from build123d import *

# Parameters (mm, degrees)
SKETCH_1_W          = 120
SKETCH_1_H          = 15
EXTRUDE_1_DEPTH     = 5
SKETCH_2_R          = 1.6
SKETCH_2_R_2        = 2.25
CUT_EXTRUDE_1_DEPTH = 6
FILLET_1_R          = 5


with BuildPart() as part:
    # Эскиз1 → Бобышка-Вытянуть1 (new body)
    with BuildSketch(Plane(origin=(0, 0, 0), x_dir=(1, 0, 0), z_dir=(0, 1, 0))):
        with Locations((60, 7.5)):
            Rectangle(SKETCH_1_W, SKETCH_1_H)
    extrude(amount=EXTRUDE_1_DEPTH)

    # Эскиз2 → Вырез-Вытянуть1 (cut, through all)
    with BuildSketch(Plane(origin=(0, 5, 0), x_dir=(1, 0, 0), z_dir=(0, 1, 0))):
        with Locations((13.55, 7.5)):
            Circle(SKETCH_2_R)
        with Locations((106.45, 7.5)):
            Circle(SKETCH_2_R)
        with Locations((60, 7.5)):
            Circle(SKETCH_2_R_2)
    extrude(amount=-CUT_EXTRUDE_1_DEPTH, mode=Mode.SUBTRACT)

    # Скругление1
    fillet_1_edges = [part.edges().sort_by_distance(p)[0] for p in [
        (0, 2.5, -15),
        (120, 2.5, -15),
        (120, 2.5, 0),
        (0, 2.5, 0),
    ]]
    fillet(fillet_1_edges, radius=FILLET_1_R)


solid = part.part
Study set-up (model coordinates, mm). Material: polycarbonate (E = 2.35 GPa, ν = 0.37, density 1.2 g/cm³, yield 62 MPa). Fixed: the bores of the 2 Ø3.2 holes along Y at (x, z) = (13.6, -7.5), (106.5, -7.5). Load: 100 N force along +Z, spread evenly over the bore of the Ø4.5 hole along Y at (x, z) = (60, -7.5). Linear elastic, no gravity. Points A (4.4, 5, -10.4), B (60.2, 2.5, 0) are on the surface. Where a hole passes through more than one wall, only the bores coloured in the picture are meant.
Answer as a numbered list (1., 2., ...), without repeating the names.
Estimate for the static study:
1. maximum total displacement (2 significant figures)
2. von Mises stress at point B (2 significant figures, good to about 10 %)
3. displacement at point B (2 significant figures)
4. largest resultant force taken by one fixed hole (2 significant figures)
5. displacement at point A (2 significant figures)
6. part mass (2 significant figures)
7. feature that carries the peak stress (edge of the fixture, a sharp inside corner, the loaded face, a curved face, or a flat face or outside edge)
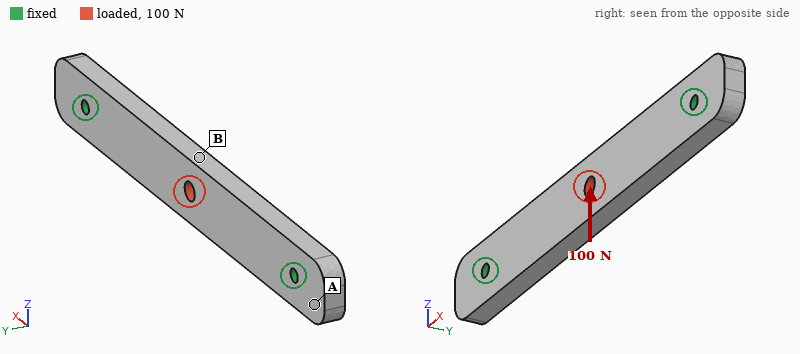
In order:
1. 0.29 mm
2. 8.4 MPa
3. 0.28 mm
4. 50 N
5. 0.047 mm
6. 10 g
7. edge of the fixture
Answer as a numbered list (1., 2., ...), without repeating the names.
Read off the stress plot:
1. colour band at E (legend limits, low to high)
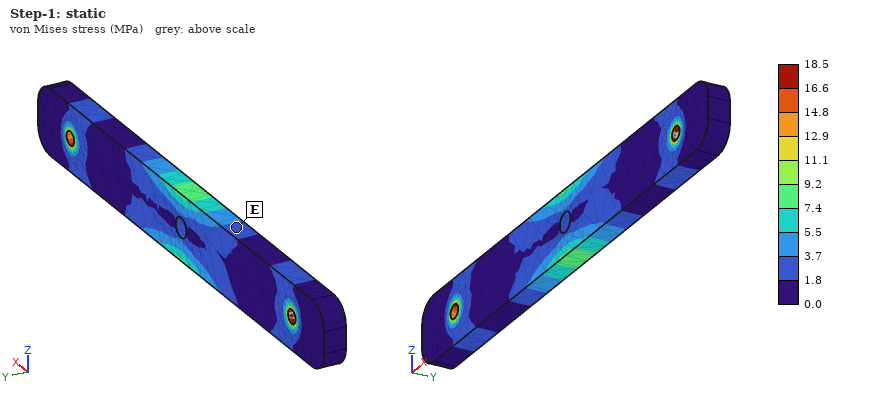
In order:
1. 1.8 to 3.7 MPa
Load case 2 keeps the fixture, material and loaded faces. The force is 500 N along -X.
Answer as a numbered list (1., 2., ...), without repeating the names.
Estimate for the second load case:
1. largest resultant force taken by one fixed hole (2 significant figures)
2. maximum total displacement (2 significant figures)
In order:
1. 250 N
2. 76 µm
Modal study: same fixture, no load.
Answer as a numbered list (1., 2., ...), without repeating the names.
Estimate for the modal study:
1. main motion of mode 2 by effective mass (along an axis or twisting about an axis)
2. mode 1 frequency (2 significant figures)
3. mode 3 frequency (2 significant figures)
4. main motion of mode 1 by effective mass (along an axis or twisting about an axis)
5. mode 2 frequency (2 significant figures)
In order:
1. along Z
2. 810 Hz
3. 2200 Hz
4. along Y
5. 1500 Hz
